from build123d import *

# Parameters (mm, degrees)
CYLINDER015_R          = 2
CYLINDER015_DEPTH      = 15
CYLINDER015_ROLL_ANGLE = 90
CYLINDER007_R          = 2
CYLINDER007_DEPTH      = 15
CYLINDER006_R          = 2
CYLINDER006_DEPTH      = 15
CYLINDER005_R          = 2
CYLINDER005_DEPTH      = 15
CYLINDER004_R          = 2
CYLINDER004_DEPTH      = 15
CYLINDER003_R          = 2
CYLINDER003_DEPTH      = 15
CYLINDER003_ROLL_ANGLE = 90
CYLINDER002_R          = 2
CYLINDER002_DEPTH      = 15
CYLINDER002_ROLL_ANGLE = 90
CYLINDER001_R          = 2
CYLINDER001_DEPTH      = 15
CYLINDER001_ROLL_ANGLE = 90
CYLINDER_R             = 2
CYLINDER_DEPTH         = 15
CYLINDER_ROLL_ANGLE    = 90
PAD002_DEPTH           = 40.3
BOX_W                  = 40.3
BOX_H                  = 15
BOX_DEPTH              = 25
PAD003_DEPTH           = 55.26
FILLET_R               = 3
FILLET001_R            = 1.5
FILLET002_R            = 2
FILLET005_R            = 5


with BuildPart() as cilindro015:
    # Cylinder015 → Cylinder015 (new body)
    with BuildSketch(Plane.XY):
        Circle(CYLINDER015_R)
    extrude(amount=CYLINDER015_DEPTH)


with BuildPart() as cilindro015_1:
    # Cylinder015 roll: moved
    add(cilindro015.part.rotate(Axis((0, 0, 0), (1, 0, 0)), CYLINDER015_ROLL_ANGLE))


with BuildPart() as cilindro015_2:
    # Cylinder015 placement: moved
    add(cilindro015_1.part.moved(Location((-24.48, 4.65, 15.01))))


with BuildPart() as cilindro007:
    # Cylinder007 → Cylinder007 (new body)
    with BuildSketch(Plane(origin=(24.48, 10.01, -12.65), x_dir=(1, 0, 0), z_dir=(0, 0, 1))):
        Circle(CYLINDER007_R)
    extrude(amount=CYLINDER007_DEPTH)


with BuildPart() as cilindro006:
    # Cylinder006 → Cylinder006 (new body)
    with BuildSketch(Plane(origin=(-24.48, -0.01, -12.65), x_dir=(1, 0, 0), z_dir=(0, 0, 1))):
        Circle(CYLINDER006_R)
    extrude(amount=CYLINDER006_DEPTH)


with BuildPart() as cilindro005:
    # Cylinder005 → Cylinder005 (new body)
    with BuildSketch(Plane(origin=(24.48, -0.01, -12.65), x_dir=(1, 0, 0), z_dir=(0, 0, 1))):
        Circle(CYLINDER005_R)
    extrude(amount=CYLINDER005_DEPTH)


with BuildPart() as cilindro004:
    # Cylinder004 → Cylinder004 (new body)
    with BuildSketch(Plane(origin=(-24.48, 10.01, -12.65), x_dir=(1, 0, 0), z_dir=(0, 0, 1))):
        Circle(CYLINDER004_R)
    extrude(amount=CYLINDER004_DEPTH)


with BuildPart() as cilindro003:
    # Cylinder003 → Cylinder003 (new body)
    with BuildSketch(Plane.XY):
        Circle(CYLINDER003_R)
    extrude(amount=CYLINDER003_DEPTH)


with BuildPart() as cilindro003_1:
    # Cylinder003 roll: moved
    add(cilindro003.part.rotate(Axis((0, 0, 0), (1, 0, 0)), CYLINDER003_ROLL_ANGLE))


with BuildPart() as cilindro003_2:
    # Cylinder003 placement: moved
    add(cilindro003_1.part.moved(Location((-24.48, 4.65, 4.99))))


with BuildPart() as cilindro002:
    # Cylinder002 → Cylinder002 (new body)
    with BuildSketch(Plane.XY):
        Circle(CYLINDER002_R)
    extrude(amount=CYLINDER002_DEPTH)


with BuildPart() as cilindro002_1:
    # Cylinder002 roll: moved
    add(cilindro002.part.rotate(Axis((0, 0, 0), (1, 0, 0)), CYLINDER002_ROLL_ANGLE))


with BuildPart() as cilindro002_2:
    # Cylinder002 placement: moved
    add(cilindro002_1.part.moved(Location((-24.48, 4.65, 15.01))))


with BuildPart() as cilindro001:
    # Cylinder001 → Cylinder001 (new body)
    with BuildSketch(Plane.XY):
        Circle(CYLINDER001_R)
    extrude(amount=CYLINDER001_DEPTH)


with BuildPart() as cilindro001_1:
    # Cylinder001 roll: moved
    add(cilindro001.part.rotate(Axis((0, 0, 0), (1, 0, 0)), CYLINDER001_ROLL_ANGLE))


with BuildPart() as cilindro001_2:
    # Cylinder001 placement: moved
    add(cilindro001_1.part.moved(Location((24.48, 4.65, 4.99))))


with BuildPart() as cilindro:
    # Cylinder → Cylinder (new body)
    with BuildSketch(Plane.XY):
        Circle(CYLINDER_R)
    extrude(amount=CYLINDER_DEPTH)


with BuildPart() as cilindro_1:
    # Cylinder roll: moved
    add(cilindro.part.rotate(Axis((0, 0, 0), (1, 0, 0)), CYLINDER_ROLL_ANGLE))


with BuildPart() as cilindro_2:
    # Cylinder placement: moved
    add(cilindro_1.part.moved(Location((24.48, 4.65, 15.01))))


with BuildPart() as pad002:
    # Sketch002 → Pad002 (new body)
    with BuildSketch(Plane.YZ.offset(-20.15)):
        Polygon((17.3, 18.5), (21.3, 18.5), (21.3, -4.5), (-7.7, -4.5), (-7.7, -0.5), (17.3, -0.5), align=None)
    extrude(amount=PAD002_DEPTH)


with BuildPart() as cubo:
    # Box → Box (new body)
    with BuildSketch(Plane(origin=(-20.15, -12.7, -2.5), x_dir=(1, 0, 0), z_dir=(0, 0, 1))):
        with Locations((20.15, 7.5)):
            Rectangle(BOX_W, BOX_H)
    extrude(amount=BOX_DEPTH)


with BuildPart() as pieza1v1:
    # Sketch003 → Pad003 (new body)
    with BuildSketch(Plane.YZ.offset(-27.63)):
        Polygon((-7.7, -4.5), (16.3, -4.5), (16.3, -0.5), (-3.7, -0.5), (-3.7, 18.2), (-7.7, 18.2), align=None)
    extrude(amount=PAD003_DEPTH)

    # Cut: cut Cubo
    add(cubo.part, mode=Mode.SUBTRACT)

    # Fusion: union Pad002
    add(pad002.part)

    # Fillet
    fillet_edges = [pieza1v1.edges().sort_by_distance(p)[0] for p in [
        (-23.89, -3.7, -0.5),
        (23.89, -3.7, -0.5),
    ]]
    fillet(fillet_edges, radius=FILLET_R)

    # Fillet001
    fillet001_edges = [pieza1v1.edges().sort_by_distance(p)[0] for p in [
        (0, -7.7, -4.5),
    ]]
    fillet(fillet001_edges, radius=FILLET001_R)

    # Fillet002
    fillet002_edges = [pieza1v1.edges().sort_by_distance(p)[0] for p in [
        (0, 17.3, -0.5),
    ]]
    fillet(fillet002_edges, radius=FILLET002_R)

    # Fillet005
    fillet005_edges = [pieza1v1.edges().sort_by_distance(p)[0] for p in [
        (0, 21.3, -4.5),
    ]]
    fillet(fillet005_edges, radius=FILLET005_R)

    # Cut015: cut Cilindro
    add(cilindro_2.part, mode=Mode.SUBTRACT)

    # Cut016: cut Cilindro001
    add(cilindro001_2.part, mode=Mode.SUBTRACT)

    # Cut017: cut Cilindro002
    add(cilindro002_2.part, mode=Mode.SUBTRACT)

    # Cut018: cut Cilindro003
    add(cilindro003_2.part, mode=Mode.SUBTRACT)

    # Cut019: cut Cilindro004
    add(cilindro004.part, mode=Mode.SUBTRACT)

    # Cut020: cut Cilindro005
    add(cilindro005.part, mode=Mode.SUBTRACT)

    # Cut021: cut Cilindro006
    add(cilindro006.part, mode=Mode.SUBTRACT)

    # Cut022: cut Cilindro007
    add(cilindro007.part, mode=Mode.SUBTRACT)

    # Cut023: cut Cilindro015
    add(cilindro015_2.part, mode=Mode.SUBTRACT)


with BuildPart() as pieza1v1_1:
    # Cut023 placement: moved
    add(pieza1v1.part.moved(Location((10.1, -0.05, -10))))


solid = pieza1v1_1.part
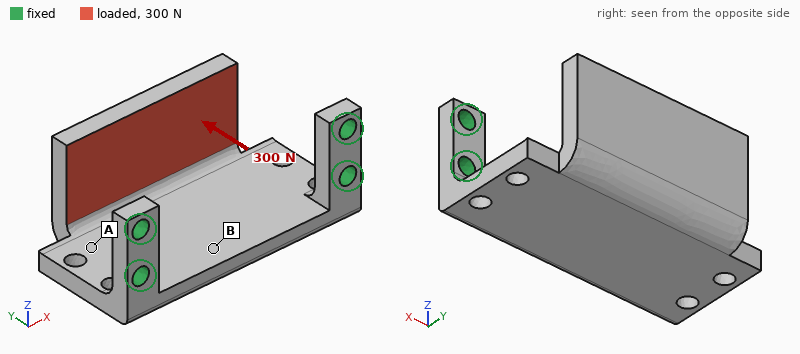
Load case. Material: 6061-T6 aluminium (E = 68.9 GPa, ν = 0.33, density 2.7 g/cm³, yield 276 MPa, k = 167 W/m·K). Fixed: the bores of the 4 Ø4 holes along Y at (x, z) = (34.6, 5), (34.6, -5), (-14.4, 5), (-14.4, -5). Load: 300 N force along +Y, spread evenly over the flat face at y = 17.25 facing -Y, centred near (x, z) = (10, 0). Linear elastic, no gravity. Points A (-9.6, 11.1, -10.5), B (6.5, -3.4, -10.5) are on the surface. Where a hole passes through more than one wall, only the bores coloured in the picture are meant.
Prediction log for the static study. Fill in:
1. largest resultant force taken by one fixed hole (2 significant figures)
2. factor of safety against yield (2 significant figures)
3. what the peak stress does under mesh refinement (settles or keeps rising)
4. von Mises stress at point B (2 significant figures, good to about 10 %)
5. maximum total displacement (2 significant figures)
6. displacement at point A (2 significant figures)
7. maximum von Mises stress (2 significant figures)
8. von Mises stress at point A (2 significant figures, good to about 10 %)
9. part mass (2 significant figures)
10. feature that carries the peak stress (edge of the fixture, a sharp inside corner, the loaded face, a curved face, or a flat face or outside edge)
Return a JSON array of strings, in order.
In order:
["150 N", "2.0", "settles", "8.9 MPa", "0.25 mm", "0.078 mm", "140 MPa", "31 MPa", "26 g", "a curved face"]
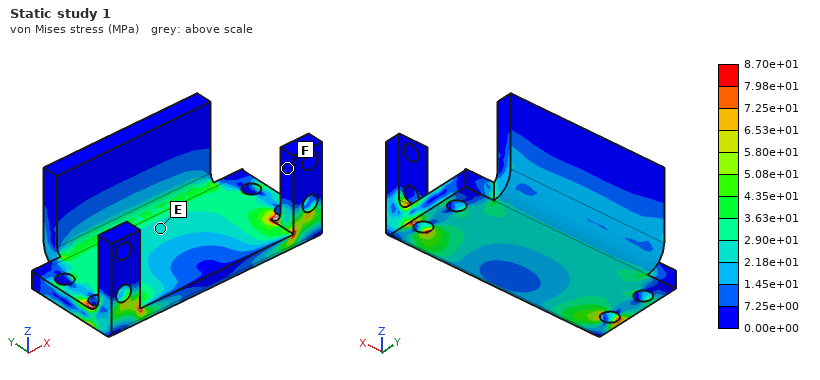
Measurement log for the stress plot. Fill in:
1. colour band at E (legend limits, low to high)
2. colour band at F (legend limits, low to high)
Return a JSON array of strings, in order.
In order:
["2.18e+01 to 2.90e+01 MPa", "0.00e+00 to 7.25e+00 MPa"]
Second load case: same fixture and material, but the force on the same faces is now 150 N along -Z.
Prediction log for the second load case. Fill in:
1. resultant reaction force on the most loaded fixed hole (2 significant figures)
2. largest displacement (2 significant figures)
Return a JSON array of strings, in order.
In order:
["78 N", "0.18 mm"]
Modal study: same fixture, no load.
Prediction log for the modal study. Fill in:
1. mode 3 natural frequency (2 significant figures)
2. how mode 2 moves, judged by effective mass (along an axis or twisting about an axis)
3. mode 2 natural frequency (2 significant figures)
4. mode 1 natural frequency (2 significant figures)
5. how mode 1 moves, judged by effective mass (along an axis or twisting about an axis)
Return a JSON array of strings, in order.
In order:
["4600 Hz", "along X", "3400 Hz", "1300 Hz", "along Z"]
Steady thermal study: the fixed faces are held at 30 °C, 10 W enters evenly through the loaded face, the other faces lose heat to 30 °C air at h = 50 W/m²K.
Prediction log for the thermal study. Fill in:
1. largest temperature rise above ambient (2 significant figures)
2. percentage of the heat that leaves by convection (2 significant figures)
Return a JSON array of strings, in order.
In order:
["17 K", "24 %"]
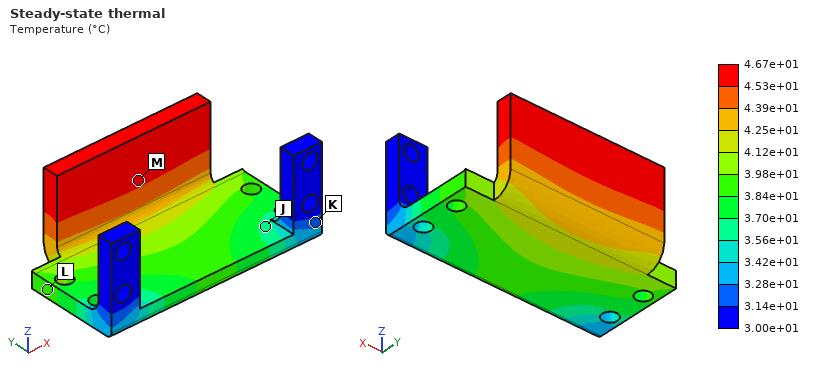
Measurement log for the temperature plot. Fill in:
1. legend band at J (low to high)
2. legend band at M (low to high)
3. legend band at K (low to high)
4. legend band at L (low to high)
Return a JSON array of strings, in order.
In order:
["3.56e+01 to 3.70e+01 °C", "4.53e+01 to 4.67e+01 °C", "3.14e+01 to 3.28e+01 °C", "3.84e+01 to 3.98e+01 °C"]
